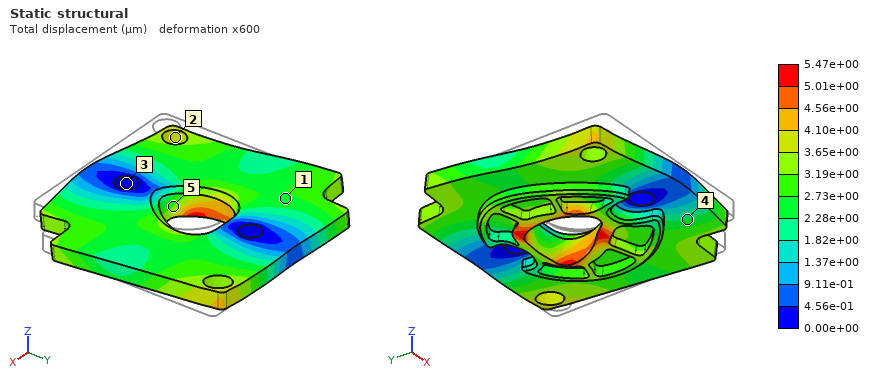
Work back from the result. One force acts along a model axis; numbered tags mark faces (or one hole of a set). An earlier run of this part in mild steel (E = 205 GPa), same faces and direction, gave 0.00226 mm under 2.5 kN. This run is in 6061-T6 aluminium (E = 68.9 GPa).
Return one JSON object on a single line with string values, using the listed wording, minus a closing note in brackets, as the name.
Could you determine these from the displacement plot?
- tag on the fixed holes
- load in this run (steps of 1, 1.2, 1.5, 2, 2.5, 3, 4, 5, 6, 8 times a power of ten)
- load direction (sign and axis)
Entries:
{"tag on the fixed holes": "3", "load in this run": "2 kN", "load direction": "+Y"}
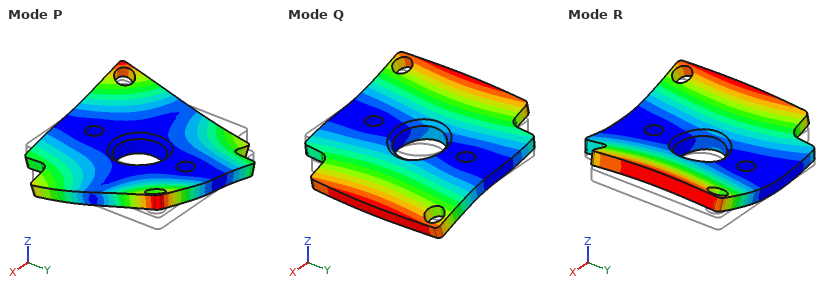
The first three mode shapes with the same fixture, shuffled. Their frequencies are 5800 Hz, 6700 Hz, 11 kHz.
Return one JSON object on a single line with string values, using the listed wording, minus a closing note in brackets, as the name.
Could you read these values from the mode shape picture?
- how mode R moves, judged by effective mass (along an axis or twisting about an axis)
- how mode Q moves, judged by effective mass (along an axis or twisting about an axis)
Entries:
{"how mode R moves, judged by effective mass": "along Z", "how mode Q moves, judged by effective mass": "twisting about Y"}
